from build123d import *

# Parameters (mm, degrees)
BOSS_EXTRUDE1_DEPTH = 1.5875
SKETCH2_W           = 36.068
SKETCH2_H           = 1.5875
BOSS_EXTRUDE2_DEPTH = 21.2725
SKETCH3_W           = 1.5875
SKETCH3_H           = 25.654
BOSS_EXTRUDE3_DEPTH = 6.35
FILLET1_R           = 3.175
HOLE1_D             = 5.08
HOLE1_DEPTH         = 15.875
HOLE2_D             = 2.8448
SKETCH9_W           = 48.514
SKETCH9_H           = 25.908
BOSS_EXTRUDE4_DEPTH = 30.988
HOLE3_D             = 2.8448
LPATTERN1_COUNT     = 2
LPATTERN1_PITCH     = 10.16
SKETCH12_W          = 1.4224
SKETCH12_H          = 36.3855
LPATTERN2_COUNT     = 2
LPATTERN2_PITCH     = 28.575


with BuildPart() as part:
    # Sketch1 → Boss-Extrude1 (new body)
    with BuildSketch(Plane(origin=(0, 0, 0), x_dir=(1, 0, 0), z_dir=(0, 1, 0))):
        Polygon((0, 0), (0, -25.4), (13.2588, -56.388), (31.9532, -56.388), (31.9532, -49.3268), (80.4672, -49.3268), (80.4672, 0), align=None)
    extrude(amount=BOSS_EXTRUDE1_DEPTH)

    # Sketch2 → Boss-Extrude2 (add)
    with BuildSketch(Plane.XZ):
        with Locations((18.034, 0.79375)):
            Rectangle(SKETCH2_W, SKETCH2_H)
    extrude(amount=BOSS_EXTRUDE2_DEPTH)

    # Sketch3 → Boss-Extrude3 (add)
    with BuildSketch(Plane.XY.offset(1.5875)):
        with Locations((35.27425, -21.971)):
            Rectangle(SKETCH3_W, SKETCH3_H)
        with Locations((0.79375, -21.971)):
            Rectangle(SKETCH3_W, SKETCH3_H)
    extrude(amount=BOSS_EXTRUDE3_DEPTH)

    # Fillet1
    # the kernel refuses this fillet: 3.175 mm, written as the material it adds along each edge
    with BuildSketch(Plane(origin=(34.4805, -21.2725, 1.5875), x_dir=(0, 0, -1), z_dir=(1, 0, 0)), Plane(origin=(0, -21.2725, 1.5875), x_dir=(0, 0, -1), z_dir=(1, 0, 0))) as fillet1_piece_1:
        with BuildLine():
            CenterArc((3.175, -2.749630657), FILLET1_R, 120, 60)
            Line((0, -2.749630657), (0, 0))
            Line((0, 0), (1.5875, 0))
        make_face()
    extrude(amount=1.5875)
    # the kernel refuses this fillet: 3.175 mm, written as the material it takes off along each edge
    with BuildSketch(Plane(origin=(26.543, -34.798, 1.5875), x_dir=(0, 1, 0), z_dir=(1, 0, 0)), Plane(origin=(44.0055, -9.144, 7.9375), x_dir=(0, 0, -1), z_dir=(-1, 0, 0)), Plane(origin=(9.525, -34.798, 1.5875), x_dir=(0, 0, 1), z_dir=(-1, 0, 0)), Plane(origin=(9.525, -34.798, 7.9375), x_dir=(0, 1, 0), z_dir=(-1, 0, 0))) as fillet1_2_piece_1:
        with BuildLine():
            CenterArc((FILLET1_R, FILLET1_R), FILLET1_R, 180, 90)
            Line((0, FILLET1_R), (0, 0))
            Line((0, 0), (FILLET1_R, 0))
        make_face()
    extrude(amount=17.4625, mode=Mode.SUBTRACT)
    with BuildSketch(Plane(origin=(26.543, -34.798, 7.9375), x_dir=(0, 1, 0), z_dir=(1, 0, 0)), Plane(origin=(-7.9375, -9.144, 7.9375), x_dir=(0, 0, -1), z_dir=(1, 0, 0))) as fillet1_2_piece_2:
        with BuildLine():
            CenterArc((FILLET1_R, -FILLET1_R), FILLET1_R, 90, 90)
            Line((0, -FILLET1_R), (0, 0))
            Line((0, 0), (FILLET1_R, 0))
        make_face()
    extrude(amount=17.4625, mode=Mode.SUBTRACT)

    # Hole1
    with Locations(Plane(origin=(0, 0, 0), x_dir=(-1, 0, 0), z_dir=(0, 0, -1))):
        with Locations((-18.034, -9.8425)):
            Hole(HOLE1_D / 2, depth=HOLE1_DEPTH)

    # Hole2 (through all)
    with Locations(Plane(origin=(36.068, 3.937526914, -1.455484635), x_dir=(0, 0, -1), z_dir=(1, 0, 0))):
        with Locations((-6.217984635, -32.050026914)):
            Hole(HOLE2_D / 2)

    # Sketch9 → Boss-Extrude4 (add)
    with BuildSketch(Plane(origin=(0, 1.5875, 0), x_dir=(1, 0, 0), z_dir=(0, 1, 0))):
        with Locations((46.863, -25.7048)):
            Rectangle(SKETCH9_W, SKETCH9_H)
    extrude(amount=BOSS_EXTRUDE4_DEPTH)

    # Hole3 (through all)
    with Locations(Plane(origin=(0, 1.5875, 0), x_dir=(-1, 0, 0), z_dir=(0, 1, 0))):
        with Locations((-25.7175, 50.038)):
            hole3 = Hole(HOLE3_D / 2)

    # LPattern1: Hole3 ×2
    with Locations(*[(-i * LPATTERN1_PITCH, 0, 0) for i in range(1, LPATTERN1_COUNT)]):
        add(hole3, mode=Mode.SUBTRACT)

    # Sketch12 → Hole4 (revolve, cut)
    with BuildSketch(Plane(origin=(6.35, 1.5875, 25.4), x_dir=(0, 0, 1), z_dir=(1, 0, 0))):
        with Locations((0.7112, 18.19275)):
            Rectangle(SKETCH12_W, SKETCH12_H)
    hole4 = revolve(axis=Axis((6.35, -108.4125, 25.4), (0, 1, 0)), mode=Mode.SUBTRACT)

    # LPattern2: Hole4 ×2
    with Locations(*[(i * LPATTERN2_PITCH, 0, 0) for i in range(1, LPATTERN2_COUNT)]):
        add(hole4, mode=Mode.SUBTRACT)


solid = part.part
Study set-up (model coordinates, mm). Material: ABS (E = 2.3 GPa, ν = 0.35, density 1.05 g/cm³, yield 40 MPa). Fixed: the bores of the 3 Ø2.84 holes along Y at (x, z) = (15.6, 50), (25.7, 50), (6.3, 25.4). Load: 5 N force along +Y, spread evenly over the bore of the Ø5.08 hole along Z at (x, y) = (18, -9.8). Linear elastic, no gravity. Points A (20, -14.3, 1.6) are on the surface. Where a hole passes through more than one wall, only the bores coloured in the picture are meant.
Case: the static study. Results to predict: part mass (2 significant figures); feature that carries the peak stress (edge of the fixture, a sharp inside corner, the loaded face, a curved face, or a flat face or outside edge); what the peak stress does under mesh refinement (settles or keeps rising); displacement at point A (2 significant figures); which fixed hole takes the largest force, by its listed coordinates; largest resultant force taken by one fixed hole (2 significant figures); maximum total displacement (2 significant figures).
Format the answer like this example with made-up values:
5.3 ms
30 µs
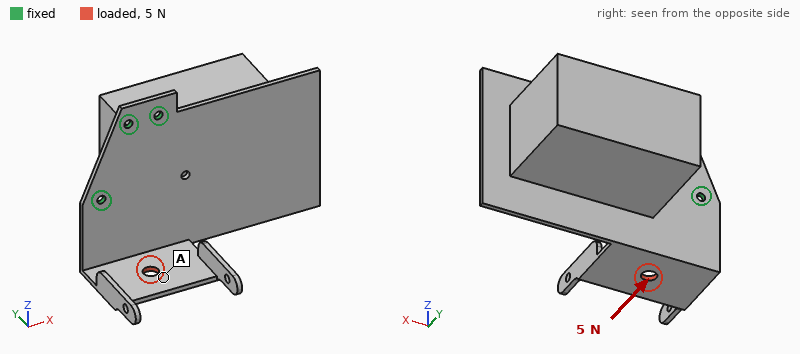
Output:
49 g
edge of the fixture
keeps rising
0.88 mm
(6.3, 25.4)
7.5 N
1.4 mm
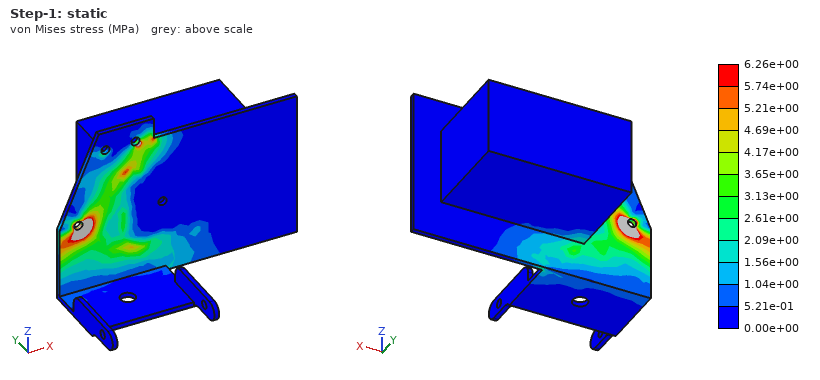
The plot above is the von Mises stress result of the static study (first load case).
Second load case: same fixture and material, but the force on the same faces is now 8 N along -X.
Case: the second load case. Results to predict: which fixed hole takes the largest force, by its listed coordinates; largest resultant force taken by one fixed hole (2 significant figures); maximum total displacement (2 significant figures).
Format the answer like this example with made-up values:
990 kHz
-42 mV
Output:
(6.3, 25.4)
13 N
1.2 mm
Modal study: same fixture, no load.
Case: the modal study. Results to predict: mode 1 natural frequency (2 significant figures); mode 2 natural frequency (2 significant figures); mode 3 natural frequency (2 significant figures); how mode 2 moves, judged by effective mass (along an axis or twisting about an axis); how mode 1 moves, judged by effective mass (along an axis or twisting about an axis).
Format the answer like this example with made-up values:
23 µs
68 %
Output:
43 Hz
160 Hz
280 Hz
along Z
along Y
